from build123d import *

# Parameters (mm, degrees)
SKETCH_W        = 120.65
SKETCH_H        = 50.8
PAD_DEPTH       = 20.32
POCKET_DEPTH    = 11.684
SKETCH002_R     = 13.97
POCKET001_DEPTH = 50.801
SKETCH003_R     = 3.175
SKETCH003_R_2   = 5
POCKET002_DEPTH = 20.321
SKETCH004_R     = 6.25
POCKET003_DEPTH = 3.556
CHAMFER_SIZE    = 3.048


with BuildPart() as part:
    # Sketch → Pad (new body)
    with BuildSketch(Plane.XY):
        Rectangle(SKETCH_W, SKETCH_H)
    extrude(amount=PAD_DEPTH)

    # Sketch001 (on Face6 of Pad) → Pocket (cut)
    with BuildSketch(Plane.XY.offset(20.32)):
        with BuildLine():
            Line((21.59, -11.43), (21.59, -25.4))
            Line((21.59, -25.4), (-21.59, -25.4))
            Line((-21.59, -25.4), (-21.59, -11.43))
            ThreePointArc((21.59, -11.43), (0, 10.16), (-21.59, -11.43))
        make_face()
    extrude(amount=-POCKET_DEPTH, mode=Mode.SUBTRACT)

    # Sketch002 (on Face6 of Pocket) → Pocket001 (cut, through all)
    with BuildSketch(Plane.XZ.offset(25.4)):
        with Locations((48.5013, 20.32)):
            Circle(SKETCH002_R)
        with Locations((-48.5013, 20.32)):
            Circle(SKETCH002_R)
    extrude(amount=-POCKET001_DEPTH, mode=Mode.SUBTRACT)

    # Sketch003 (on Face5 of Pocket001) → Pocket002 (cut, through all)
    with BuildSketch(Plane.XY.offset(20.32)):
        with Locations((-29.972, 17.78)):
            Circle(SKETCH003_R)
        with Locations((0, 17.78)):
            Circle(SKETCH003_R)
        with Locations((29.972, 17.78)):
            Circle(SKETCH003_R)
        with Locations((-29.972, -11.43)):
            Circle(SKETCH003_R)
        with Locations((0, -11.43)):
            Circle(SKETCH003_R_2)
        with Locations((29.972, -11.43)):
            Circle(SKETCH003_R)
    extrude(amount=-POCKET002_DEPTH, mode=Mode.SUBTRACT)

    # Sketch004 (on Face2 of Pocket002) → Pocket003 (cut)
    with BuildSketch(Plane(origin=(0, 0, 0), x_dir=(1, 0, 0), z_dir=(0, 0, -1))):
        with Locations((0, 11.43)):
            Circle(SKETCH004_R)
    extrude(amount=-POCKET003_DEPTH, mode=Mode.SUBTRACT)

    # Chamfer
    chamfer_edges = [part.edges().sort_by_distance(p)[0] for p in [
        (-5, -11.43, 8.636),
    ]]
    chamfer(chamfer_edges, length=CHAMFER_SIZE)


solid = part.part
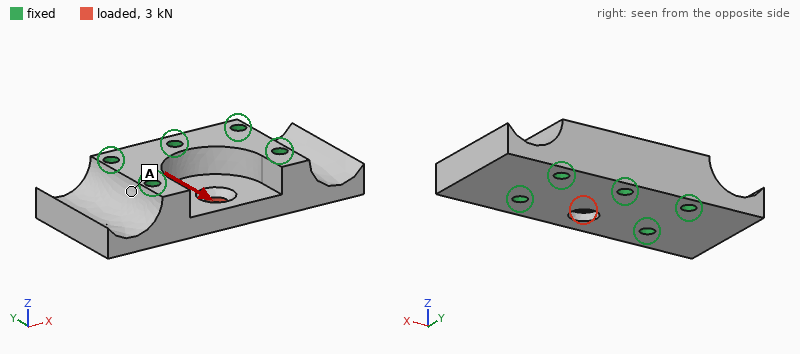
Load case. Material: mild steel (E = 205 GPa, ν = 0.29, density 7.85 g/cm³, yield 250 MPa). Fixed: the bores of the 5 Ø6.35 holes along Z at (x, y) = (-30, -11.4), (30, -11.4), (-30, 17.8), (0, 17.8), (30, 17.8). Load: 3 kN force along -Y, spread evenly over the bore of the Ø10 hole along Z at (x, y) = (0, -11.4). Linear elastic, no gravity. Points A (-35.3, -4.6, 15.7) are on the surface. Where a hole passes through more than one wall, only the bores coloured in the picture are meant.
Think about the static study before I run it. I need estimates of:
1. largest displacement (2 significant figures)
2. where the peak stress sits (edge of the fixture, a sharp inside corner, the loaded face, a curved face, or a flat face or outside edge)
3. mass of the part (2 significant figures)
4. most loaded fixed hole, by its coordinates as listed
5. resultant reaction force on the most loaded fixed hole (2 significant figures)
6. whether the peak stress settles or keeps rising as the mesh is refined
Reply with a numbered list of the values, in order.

1. 2.4 µm
2. a sharp inside corner
3. 590 g
4. (0, 17.8)
5. 1.2 kN
6. keeps rising
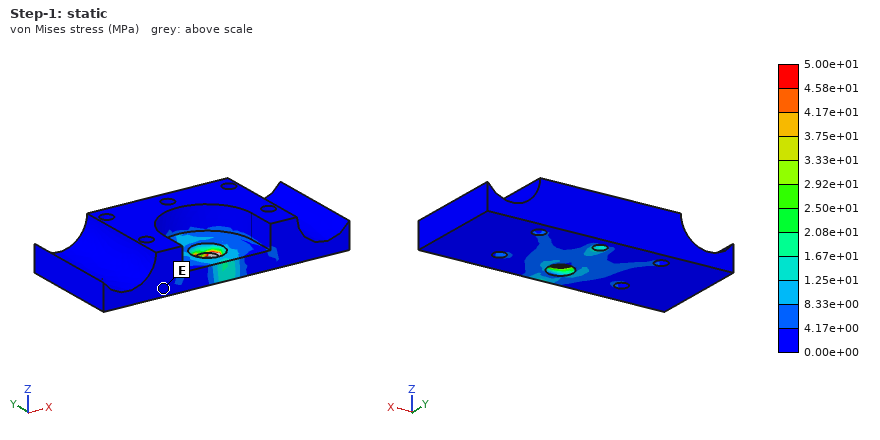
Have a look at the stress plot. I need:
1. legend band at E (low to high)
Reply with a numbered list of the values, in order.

1. 0.00e+00 to 4.17e+00 MPa
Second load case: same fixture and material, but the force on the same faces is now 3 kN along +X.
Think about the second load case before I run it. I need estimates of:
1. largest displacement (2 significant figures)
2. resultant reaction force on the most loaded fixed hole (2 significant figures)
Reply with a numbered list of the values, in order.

1. 1.6 µm
2. 1.1 kN
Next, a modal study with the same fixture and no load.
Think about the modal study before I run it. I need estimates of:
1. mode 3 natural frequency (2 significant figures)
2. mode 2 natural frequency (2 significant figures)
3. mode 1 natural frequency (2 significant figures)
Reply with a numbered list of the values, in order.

1. 13 kHz
2. 9000 Hz
3. 9000 Hz
